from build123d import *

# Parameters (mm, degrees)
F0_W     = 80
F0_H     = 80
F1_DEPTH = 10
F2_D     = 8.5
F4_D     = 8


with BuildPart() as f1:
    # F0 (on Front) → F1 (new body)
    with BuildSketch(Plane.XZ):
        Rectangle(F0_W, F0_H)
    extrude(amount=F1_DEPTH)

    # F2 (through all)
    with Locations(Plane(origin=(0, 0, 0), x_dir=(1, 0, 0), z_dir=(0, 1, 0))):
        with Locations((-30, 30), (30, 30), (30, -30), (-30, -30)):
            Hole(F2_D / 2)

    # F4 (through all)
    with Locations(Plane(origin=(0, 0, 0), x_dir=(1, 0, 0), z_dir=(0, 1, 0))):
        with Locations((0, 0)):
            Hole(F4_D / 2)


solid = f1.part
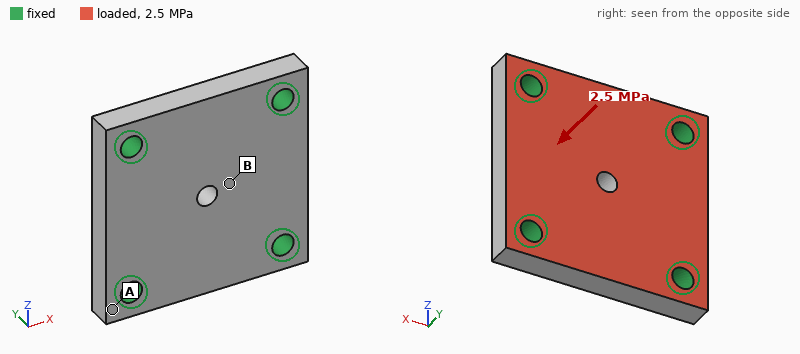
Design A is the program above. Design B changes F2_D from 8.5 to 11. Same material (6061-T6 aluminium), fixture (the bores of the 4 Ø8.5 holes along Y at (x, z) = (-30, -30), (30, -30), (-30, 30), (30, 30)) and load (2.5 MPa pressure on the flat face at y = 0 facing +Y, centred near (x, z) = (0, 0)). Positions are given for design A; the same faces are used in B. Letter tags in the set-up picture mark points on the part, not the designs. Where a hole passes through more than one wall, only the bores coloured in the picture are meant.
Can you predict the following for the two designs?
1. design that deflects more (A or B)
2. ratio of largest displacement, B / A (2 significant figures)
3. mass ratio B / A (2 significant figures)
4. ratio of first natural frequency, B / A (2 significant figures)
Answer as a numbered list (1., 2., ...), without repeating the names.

1. A
2. 0.84
3. 0.97
4. 1.1
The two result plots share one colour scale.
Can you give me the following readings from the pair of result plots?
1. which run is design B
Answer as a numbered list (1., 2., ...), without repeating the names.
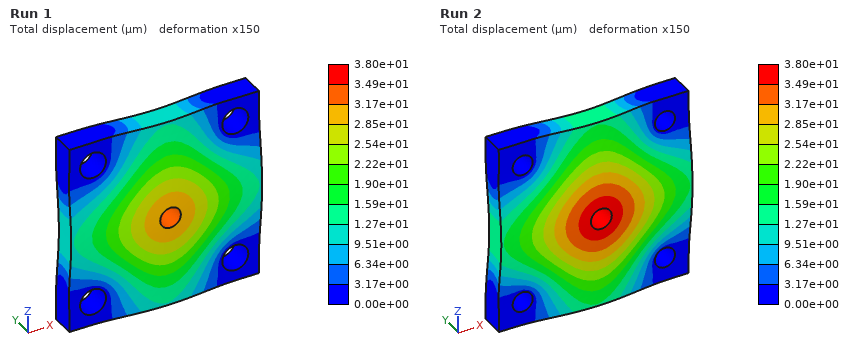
1. Run 1
